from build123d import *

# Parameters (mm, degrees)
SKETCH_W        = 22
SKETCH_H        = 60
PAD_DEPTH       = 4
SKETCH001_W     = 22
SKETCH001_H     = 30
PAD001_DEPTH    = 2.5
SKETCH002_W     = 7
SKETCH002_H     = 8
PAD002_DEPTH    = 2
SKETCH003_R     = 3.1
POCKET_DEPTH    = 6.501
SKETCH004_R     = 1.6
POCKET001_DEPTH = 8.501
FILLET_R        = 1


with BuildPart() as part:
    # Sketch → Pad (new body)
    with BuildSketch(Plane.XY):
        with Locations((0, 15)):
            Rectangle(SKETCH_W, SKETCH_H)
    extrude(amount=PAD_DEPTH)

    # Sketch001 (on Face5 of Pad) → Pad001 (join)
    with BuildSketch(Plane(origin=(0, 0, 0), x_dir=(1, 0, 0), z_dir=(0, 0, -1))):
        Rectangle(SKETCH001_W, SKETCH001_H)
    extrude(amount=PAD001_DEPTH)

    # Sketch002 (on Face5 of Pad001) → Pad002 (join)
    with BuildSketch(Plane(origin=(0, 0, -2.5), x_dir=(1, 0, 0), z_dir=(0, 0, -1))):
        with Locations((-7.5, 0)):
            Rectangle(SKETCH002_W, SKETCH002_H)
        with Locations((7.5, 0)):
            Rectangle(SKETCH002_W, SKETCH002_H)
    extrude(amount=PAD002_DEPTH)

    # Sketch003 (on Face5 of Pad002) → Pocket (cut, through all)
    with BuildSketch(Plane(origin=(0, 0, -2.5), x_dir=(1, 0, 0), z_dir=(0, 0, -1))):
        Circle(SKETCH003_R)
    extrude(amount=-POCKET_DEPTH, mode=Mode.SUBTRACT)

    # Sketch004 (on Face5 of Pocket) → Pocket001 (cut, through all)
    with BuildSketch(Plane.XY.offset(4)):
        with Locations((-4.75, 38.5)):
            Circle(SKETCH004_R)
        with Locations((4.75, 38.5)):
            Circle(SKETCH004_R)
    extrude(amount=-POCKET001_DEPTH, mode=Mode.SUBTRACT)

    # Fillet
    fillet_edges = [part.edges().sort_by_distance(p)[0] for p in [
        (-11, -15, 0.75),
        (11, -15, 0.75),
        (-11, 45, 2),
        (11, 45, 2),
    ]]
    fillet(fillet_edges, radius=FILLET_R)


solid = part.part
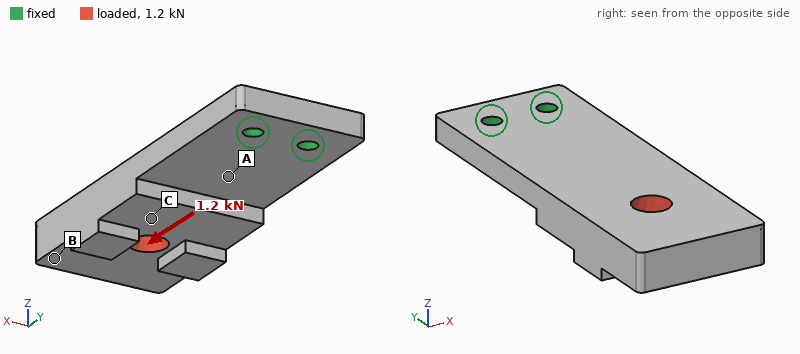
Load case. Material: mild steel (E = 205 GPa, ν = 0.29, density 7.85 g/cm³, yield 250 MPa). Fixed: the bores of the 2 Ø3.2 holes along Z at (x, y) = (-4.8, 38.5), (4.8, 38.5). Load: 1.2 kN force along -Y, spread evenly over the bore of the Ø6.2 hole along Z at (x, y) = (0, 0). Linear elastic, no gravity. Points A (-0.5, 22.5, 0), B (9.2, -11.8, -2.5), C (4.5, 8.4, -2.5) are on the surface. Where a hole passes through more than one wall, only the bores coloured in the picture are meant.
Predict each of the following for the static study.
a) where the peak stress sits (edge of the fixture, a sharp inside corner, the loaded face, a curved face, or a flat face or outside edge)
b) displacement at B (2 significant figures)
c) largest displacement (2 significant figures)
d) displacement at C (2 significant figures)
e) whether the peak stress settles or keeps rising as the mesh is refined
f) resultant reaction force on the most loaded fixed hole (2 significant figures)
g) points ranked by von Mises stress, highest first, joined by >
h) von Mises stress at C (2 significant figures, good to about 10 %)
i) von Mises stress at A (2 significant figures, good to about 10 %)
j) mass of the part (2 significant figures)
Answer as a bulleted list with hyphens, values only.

- edge of the fixture
- 56 µm
- 61 µm
- 27 µm
- keeps rising
- 600 N
- A > C > B
- 10 MPa
- 38 MPa
- 54 g
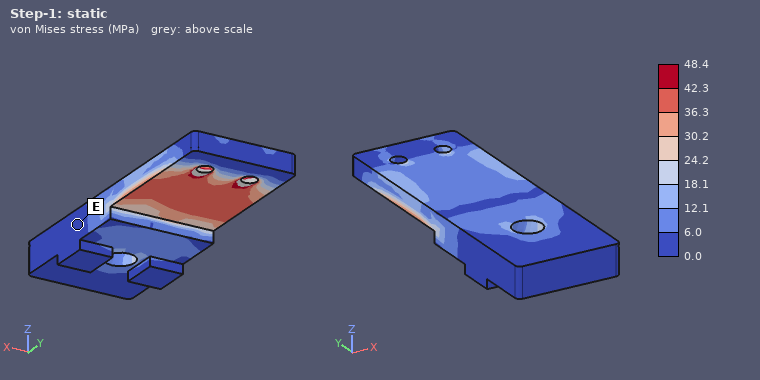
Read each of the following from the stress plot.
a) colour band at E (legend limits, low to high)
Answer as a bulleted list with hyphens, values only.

- 0.0 to 6.0 MPa
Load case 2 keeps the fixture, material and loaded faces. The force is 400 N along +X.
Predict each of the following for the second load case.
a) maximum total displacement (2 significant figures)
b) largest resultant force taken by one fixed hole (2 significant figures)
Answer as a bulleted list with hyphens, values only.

- 24 µm
- 1.3 kN
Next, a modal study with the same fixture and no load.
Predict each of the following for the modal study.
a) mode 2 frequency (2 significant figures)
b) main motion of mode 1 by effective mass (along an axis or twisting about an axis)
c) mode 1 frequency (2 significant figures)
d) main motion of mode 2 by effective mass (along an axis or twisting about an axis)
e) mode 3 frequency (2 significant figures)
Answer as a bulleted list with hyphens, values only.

- 4000 Hz
- along Z
- 950 Hz
- along X
- 4900 Hz
